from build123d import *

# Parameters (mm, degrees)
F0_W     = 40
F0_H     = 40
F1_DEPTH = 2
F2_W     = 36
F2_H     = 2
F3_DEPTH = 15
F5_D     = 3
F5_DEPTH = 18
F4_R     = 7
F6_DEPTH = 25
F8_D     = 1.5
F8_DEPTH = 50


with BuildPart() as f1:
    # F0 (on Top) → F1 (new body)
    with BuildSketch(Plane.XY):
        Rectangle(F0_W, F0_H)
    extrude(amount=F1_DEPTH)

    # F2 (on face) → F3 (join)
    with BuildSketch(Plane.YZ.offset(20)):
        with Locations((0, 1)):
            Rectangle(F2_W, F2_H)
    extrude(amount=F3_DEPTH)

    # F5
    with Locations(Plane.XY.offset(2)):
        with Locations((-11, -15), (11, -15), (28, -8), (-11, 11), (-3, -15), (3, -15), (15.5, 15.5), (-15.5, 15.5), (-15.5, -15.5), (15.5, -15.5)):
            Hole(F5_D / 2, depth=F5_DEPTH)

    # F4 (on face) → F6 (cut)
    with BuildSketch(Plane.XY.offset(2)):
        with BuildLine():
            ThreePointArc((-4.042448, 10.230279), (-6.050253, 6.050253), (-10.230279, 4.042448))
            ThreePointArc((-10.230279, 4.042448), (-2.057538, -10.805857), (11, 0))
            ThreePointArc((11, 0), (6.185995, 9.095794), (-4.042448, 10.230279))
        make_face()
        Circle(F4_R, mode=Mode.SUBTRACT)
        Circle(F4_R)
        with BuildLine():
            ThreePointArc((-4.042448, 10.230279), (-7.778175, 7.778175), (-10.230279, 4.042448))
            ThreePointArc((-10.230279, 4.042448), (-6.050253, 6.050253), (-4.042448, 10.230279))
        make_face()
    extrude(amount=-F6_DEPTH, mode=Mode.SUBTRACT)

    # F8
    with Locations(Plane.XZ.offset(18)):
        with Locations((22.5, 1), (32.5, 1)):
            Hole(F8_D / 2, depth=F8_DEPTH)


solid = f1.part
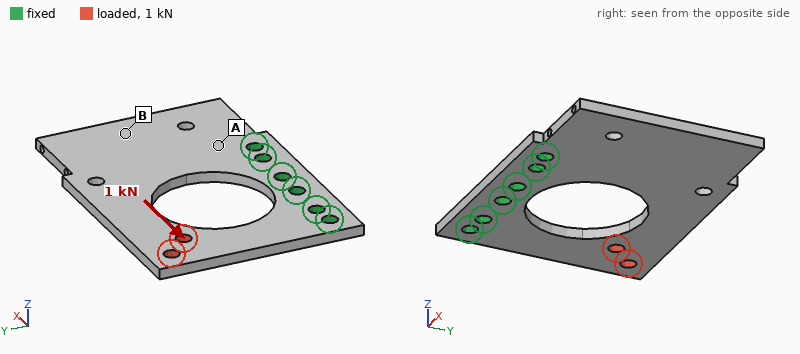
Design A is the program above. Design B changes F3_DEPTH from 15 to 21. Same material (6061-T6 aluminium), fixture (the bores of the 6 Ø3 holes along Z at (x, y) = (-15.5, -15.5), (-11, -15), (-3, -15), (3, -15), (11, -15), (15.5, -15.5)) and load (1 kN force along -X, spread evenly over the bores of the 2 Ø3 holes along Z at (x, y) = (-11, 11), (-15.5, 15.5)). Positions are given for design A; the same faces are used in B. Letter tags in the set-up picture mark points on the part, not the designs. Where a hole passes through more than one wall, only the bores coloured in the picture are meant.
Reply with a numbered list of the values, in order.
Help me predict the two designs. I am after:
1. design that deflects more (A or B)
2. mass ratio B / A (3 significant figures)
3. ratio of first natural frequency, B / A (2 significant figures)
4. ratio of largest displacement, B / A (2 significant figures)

1. B
2. 1.13
3. 0.92
4. 1.1
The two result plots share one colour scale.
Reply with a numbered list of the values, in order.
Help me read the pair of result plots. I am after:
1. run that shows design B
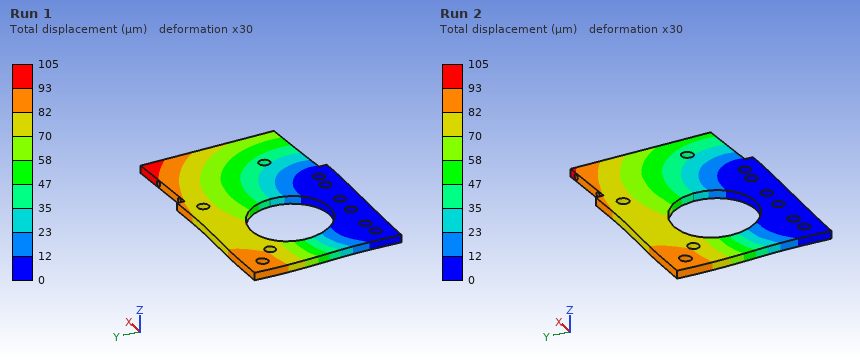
1. Run 1
